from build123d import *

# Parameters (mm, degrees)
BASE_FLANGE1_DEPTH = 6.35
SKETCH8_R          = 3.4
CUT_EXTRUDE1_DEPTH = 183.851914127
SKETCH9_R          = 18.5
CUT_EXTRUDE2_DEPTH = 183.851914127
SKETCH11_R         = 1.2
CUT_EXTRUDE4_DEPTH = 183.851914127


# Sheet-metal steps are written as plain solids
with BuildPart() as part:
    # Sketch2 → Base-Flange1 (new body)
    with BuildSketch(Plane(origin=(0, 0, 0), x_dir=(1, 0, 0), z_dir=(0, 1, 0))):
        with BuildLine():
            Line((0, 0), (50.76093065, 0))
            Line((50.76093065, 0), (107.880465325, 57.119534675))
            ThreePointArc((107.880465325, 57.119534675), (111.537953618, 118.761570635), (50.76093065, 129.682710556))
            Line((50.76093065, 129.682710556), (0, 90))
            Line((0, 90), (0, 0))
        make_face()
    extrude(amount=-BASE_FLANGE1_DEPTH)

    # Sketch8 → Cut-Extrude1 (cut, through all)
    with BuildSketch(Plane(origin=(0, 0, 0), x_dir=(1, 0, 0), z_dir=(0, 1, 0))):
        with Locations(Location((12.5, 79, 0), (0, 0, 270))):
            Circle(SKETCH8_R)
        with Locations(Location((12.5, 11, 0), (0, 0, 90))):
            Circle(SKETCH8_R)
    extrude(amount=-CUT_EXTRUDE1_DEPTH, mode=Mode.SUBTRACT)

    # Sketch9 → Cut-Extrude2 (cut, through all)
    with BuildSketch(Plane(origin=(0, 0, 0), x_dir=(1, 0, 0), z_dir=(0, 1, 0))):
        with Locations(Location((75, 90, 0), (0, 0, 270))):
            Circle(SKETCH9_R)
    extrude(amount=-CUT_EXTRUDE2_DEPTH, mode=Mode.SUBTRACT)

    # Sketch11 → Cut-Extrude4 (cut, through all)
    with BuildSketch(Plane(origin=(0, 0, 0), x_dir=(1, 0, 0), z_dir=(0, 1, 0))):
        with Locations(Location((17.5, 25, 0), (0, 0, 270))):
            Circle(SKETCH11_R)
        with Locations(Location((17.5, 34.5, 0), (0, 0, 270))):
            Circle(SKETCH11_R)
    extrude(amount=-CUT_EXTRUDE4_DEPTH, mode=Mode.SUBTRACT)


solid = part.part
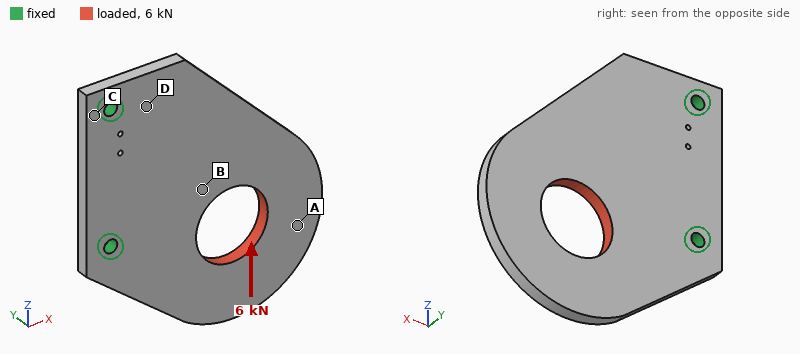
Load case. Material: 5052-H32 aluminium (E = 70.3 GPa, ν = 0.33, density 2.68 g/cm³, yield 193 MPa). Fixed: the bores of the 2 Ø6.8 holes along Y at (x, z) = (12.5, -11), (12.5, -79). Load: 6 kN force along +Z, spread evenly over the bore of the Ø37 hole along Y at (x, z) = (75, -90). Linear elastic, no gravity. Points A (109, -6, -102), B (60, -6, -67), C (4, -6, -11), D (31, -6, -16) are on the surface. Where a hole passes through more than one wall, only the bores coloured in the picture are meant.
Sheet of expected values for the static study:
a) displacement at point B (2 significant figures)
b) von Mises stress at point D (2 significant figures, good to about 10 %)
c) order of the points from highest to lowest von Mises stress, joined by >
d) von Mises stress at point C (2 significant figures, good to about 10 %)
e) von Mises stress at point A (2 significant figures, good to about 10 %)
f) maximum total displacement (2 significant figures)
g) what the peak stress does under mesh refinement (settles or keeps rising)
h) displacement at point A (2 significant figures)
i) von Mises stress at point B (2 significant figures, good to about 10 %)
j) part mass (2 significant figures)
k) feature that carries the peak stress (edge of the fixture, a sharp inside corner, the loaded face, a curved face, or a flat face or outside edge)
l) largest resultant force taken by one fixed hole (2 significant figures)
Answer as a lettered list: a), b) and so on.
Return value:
a) 0.038 mm
b) 31 MPa
c) D > B > C > A
d) 15 MPa
e) 6.8 MPa
f) 0.10 mm
g) keeps rising
h) 0.097 mm
i) 24 MPa
j) 190 g
k) edge of the fixture
l) 6.1 kN
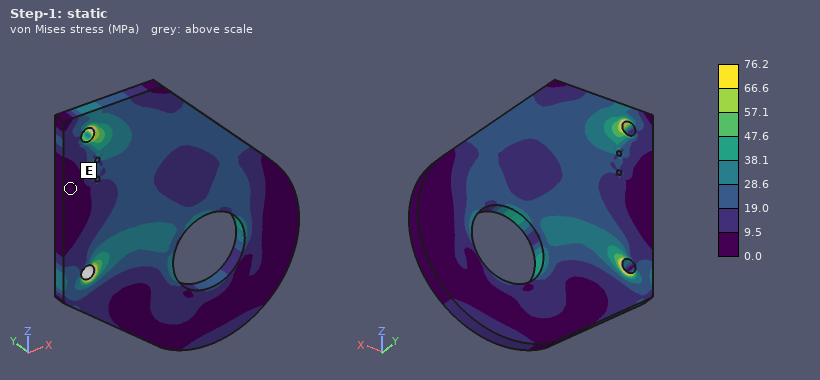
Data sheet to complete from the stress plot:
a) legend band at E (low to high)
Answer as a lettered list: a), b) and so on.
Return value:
a) 0.0 to 9.5 MPa
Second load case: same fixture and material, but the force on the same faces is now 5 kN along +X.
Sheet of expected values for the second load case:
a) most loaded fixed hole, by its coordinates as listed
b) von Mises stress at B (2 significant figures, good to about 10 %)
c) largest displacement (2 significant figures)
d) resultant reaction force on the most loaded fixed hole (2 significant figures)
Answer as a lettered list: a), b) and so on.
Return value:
a) (12.5, -79)
b) 19 MPa
c) 55 µm
d) 5.7 kN
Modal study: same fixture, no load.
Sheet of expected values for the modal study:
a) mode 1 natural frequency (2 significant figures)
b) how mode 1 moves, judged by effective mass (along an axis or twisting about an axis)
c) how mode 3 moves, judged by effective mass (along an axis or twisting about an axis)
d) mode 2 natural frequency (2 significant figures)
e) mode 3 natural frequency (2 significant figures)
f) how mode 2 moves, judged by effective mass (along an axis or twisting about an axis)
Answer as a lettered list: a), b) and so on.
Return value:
a) 480 Hz
b) along Y
c) along Y
d) 1100 Hz
e) 2200 Hz
f) twisting about X
